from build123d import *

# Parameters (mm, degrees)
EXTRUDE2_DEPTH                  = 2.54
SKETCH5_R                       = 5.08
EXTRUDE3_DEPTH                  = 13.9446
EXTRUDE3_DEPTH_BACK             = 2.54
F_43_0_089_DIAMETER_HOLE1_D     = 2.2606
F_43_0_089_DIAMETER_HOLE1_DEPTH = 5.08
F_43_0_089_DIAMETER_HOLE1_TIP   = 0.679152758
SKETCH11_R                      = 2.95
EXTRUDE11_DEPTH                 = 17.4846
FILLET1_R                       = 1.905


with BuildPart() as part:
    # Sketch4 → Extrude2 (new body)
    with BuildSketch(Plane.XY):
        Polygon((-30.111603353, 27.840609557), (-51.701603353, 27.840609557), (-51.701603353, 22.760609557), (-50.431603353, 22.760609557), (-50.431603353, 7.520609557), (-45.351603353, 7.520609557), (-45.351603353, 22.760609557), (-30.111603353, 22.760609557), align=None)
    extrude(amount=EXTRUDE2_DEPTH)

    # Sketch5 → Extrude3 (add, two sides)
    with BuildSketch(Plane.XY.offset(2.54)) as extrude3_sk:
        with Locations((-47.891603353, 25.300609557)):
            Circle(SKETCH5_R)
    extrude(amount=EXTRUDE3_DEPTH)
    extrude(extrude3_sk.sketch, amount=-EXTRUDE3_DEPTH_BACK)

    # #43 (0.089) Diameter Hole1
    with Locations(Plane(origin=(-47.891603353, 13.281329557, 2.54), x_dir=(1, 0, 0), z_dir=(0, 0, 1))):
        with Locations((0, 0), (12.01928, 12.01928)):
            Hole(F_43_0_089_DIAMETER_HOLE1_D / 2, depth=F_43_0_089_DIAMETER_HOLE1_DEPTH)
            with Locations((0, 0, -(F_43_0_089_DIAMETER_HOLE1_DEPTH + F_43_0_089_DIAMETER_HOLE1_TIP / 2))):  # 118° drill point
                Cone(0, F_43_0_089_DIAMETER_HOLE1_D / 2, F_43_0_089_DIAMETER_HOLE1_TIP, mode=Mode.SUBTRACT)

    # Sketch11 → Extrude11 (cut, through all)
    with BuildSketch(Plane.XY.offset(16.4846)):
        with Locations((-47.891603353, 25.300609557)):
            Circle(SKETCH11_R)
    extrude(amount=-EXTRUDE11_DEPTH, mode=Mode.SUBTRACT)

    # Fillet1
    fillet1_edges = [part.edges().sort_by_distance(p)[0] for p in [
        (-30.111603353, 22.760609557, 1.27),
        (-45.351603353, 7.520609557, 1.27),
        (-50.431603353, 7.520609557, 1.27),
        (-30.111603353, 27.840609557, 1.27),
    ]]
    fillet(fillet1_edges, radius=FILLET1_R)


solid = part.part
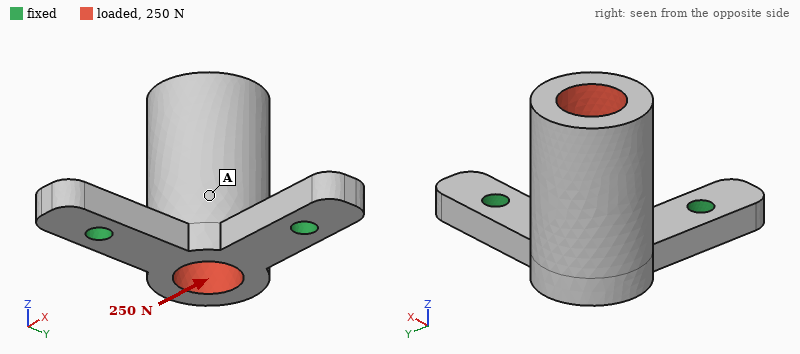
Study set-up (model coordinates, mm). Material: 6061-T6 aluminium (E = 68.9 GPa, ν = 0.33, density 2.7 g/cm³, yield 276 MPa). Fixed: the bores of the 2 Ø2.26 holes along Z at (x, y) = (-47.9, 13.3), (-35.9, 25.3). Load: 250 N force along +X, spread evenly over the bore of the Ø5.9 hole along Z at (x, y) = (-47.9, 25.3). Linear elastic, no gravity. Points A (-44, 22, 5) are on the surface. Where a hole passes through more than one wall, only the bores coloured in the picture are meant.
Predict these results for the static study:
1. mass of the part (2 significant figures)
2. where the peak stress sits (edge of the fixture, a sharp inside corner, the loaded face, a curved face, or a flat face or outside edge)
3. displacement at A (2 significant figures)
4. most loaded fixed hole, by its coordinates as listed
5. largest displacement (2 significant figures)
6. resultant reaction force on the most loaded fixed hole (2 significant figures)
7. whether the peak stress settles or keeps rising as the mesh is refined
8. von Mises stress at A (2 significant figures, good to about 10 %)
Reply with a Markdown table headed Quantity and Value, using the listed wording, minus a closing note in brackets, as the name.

| Quantity | Value |
|---|---|
| mass of the part | 3.2 g |
| where the peak stress sits | edge of the fixture |
| displacement at A | 0.037 mm |
| most loaded fixed hole, by its coordinates as listed | (-35.9, 25.3) |
| largest displacement | 0.18 mm |
| resultant reaction force on the most loaded fixed hole | 260 N |
| whether the peak stress settles or keeps rising as the mesh is refined | keeps rising |
| von Mises stress at A | 23 MPa |
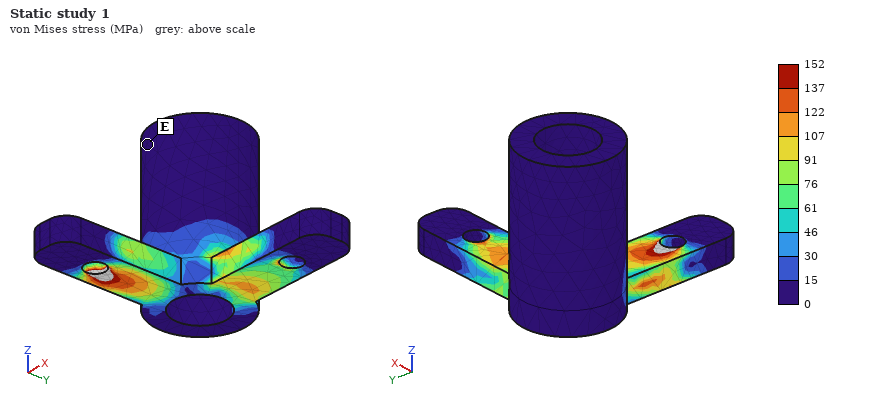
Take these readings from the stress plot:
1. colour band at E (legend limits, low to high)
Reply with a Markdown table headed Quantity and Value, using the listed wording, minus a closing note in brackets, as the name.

| Quantity | Value |
|---|---|
| colour band at E | 0 to 15 MPa |
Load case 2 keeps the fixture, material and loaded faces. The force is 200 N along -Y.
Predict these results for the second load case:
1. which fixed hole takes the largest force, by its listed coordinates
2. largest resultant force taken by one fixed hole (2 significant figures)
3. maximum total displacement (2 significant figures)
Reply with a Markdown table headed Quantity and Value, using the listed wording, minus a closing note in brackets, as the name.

| Quantity | Value |
|---|---|
| which fixed hole takes the largest force, by its listed coordinates | (-47.9, 13.3) |
| largest resultant force taken by one fixed hole | 210 N |
| maximum total displacement | 0.14 mm |
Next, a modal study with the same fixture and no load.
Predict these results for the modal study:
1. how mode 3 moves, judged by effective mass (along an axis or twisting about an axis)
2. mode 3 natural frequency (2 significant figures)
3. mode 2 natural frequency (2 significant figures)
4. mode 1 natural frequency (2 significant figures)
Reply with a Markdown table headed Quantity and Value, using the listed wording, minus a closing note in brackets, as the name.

| Quantity | Value |
|---|---|
| how mode 3 moves, judged by effective mass | along Z |
| mode 3 natural frequency | 15 kHz |
| mode 2 natural frequency | 8600 Hz |
| mode 1 natural frequency | 3500 Hz |
